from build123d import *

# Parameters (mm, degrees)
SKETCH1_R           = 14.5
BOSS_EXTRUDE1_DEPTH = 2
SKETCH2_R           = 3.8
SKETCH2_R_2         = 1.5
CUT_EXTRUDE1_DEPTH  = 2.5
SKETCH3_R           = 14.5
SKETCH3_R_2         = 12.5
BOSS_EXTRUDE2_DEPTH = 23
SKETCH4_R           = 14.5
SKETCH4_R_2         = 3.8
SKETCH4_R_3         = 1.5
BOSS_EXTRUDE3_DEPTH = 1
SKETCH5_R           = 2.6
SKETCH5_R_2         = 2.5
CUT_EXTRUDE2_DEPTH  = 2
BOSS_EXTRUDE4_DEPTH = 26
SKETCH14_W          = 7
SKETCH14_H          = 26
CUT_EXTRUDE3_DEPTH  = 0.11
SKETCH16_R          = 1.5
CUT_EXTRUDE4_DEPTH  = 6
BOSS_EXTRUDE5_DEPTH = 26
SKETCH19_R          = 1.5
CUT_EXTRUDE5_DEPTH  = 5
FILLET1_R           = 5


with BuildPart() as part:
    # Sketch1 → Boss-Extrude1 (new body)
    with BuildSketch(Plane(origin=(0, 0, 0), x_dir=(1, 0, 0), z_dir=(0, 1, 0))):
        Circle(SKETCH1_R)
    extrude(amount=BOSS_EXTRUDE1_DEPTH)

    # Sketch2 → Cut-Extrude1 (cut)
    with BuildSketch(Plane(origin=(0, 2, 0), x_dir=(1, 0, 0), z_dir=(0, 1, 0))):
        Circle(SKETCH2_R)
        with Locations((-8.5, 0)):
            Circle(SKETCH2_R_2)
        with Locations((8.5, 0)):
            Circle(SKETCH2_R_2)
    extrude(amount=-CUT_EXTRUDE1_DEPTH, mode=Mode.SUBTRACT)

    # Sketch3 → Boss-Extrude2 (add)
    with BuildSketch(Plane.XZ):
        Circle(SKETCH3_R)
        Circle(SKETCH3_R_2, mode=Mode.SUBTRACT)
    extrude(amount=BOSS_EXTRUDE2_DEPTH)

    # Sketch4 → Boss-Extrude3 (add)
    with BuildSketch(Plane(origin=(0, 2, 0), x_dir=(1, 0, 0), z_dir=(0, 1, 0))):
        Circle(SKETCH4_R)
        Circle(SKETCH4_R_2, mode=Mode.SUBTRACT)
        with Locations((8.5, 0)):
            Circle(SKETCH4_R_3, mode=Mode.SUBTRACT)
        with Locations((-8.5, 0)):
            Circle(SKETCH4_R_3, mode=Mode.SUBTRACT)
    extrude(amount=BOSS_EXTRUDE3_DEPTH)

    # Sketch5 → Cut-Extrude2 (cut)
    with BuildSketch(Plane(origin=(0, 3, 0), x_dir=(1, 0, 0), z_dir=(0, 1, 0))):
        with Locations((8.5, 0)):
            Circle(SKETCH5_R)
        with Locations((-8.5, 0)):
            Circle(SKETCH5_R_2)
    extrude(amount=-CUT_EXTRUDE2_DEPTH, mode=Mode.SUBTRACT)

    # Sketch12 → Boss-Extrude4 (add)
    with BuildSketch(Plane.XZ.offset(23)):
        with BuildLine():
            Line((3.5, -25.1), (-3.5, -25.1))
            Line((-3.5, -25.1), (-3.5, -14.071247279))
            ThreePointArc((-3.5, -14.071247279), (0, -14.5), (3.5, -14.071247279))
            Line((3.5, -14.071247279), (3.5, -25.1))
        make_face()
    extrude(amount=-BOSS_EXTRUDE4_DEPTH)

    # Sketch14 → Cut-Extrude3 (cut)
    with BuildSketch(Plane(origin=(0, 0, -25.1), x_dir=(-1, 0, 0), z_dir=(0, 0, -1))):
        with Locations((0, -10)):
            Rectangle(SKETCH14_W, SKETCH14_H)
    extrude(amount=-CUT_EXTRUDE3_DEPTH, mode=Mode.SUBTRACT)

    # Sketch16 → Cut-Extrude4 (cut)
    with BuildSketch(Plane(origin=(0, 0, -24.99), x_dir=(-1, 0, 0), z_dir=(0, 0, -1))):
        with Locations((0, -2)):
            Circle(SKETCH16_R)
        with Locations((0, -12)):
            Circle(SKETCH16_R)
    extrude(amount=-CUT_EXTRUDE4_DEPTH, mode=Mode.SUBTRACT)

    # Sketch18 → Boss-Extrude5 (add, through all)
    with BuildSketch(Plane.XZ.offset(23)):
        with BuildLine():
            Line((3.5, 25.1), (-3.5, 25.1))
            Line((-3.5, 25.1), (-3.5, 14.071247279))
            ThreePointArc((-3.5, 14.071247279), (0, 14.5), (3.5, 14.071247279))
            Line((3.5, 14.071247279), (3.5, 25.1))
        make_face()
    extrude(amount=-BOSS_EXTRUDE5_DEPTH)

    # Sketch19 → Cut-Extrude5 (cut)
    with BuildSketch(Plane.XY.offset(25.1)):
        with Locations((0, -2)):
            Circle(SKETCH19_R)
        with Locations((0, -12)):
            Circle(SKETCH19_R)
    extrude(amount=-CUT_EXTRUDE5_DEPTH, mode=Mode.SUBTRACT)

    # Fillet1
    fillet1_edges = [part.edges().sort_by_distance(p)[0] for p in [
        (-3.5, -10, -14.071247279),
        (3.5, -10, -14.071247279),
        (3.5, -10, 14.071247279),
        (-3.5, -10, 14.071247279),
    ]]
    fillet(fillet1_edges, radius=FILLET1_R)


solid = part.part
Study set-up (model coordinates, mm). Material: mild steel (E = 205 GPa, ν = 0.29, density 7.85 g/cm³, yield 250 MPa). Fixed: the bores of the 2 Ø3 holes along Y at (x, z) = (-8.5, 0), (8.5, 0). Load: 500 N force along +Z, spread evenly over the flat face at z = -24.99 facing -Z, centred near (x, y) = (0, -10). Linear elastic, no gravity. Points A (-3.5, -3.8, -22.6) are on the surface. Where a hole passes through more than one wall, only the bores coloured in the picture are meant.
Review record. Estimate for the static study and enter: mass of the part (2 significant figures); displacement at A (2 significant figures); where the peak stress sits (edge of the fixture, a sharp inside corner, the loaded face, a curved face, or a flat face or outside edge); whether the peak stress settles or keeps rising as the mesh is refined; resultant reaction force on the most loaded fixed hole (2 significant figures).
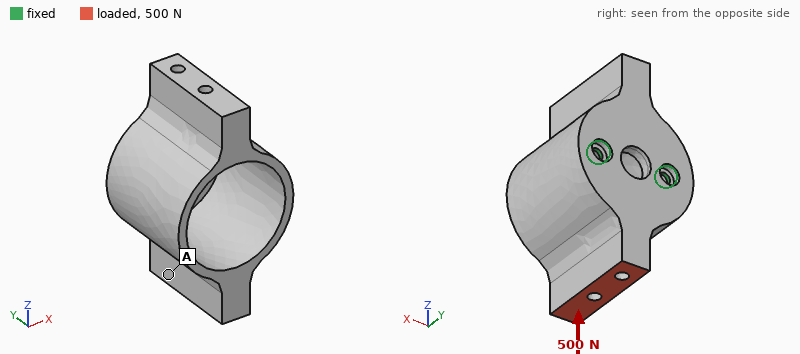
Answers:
75 g
0.091 mm
edge of the fixture
keeps rising
260 N
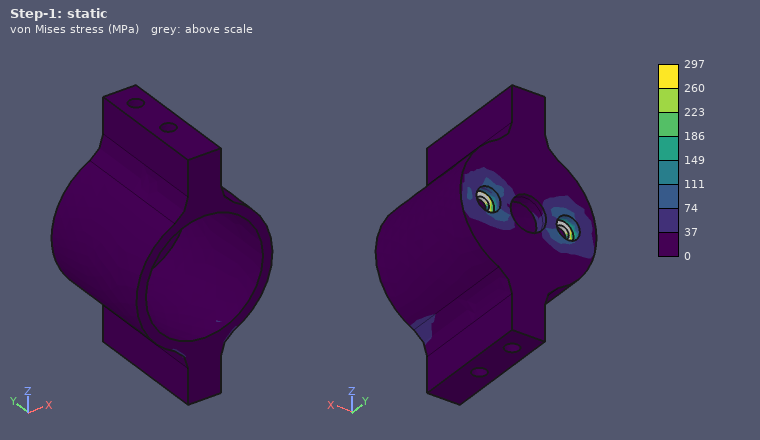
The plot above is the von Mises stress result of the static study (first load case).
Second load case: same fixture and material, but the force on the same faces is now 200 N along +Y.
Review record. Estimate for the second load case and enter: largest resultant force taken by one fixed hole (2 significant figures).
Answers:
100 N
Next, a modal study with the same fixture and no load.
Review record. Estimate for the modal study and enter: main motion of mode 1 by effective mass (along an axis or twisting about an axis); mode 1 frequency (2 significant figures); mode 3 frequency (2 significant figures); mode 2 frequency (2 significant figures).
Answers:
along Z
1200 Hz
5600 Hz
5500 Hz
